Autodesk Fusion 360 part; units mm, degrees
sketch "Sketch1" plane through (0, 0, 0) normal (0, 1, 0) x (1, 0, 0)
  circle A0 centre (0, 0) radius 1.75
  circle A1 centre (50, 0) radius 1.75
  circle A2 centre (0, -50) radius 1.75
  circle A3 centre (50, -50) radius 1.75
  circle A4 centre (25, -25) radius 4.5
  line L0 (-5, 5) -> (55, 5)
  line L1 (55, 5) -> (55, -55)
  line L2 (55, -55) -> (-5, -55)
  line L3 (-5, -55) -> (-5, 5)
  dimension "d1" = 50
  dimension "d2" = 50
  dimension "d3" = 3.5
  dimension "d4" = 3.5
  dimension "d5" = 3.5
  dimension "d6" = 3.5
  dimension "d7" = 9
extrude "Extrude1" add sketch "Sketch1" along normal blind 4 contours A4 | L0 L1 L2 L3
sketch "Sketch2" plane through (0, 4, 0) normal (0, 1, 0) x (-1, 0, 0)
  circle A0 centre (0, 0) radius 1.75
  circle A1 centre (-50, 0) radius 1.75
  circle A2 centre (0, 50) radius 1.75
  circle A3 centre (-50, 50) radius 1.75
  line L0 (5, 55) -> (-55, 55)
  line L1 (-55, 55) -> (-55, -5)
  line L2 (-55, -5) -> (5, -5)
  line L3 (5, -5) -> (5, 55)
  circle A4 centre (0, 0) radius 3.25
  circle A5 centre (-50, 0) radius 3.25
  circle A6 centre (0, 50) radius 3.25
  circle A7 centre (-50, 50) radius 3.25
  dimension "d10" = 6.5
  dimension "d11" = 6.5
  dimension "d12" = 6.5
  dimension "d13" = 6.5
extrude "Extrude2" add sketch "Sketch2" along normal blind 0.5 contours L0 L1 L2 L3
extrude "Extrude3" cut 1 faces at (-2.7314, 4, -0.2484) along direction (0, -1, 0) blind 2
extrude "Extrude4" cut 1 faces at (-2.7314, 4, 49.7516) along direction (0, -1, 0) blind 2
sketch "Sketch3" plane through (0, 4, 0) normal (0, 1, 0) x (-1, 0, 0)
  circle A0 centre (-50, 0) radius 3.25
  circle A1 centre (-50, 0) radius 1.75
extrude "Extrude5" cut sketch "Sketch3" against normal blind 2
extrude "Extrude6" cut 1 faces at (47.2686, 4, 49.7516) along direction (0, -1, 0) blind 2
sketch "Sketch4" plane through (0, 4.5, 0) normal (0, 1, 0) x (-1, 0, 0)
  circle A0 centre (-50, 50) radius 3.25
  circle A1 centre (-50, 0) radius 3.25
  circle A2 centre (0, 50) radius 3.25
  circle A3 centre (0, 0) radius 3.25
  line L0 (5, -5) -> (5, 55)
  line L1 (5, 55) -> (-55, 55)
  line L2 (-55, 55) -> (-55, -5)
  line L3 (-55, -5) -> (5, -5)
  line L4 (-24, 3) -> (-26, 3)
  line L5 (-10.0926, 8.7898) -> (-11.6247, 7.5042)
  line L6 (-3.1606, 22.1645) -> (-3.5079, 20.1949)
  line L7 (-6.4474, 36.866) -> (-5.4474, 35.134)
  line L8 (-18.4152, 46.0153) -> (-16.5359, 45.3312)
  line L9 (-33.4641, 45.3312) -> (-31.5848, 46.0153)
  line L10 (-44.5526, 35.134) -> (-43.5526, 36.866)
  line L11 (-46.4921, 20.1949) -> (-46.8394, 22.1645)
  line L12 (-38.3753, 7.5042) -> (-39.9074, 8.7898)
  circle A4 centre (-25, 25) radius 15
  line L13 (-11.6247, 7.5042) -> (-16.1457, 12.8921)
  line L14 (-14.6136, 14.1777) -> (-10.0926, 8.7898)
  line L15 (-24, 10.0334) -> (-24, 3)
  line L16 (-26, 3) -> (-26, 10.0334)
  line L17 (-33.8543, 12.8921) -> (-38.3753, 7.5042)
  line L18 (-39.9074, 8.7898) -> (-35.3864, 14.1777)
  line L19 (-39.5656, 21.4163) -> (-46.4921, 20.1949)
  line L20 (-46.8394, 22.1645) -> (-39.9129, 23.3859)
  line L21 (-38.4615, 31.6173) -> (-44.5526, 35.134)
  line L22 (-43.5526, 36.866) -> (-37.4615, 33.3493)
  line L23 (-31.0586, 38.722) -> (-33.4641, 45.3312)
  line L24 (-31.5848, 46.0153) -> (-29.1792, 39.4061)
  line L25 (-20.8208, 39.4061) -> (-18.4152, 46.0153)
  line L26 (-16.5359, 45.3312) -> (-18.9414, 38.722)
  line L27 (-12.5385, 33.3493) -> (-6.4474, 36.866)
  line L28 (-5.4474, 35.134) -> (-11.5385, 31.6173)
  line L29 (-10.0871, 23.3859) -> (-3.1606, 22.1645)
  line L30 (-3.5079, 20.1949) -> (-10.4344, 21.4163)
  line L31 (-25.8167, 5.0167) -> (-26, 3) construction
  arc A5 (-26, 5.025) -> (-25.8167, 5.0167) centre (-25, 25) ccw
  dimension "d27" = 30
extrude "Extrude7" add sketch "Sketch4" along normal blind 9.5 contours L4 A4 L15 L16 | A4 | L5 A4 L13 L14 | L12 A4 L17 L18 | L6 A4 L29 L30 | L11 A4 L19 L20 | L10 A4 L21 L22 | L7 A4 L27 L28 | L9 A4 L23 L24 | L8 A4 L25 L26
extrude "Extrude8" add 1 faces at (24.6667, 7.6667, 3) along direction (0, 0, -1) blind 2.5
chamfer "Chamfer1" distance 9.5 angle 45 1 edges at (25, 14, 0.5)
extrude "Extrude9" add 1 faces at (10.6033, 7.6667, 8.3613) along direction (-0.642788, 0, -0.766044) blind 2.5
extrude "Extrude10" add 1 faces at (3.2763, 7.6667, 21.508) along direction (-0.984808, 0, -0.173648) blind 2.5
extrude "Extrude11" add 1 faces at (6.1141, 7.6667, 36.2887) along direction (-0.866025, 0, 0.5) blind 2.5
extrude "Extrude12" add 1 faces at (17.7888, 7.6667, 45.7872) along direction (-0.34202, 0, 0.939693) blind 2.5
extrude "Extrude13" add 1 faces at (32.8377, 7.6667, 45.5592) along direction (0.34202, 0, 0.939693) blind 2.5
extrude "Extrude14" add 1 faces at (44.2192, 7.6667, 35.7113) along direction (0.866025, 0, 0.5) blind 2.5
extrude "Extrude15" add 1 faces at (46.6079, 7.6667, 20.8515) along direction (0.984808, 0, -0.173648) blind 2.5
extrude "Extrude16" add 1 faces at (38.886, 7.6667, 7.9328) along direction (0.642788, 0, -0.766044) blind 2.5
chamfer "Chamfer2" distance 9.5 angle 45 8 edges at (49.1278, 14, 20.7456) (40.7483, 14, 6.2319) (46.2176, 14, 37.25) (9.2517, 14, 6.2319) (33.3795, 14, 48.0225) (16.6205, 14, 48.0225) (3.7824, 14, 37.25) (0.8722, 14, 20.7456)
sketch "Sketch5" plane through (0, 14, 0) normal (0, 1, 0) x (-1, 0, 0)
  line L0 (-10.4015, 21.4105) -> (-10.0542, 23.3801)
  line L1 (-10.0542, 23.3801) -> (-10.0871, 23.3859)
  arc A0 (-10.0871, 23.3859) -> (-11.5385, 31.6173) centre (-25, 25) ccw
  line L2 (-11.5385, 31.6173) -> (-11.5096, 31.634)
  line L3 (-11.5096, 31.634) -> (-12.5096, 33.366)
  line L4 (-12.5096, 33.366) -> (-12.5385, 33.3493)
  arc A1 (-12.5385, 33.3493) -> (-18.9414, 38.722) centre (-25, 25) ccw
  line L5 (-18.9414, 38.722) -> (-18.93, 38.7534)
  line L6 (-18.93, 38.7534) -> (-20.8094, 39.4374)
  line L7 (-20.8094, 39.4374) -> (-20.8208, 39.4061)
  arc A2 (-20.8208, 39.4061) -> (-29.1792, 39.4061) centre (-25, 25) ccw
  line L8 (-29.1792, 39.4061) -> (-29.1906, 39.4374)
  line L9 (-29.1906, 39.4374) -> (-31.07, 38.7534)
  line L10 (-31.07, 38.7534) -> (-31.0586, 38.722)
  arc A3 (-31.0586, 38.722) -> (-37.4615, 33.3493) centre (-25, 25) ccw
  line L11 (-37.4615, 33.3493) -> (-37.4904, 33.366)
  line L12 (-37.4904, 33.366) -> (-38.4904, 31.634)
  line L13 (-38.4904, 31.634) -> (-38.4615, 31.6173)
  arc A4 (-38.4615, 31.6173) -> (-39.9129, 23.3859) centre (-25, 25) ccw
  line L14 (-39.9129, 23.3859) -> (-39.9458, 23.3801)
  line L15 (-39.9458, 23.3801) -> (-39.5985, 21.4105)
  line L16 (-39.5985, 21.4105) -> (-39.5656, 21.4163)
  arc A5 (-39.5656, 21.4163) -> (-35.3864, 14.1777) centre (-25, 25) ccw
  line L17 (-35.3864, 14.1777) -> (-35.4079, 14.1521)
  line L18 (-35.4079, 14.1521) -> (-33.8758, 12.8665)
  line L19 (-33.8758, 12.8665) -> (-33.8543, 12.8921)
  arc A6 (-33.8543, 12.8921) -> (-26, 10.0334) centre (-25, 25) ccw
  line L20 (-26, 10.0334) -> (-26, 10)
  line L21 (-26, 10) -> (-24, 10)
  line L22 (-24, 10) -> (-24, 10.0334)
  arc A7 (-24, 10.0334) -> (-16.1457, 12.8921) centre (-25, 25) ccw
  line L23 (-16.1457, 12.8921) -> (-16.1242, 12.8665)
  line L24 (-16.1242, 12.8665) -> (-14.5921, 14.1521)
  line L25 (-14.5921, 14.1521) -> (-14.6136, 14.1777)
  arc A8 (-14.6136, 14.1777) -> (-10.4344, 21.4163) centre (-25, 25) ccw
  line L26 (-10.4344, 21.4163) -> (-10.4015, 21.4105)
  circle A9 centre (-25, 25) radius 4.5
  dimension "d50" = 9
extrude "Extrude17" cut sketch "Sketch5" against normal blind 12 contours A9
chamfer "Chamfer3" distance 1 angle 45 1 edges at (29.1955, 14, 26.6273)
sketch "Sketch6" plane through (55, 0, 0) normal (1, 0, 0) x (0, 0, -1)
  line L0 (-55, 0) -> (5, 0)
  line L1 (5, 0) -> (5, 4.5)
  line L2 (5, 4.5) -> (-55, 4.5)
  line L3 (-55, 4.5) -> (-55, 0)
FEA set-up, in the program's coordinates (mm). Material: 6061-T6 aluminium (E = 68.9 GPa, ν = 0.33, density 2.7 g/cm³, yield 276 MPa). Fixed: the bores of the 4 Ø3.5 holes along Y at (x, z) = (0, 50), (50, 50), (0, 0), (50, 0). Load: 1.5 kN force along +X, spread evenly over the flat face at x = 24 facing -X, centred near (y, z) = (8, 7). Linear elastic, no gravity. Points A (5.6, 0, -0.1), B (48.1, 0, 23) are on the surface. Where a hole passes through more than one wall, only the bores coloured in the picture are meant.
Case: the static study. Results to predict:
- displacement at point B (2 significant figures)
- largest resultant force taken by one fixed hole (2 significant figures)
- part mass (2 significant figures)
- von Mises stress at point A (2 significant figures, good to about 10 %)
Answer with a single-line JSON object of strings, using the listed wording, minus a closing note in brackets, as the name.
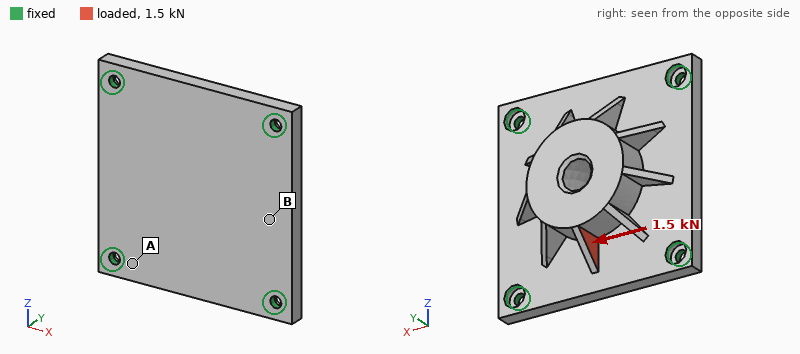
{"displacement at point B": "6.1 µm", "largest resultant force taken by one fixed hole": "560 N", "part mass": "61 g", "von Mises stress at point A": "19 MPa"}
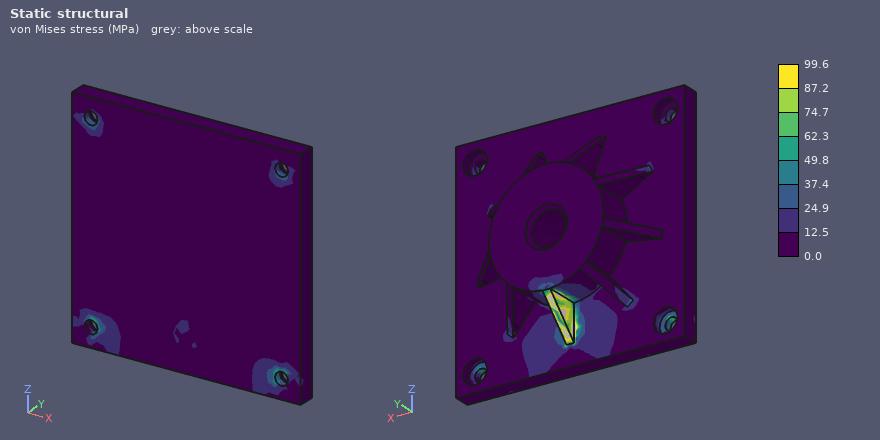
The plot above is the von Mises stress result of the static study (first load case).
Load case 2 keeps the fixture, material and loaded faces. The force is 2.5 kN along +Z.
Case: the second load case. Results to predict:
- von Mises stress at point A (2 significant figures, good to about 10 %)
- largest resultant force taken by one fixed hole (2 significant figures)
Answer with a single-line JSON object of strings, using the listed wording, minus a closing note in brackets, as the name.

{"von Mises stress at point A": "11 MPa", "largest resultant force taken by one fixed hole": "750 N"}
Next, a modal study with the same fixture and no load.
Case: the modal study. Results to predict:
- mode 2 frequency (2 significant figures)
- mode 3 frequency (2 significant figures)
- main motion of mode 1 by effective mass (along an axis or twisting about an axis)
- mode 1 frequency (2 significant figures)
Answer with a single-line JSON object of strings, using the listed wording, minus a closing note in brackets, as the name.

{"mode 2 frequency": "8300 Hz", "mode 3 frequency": "8300 Hz", "main motion of mode 1 by effective mass": "along Y", "mode 1 frequency": "5100 Hz"}
